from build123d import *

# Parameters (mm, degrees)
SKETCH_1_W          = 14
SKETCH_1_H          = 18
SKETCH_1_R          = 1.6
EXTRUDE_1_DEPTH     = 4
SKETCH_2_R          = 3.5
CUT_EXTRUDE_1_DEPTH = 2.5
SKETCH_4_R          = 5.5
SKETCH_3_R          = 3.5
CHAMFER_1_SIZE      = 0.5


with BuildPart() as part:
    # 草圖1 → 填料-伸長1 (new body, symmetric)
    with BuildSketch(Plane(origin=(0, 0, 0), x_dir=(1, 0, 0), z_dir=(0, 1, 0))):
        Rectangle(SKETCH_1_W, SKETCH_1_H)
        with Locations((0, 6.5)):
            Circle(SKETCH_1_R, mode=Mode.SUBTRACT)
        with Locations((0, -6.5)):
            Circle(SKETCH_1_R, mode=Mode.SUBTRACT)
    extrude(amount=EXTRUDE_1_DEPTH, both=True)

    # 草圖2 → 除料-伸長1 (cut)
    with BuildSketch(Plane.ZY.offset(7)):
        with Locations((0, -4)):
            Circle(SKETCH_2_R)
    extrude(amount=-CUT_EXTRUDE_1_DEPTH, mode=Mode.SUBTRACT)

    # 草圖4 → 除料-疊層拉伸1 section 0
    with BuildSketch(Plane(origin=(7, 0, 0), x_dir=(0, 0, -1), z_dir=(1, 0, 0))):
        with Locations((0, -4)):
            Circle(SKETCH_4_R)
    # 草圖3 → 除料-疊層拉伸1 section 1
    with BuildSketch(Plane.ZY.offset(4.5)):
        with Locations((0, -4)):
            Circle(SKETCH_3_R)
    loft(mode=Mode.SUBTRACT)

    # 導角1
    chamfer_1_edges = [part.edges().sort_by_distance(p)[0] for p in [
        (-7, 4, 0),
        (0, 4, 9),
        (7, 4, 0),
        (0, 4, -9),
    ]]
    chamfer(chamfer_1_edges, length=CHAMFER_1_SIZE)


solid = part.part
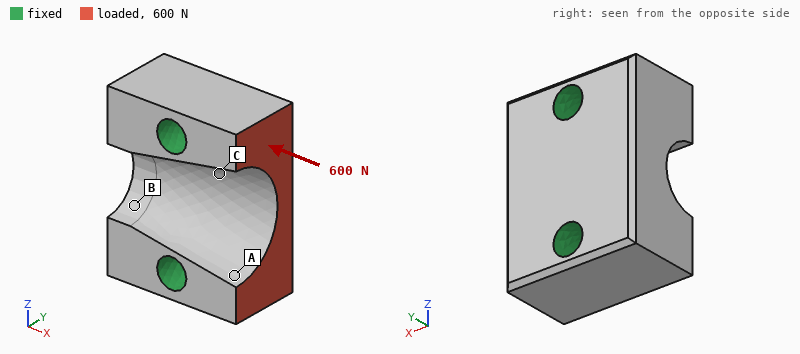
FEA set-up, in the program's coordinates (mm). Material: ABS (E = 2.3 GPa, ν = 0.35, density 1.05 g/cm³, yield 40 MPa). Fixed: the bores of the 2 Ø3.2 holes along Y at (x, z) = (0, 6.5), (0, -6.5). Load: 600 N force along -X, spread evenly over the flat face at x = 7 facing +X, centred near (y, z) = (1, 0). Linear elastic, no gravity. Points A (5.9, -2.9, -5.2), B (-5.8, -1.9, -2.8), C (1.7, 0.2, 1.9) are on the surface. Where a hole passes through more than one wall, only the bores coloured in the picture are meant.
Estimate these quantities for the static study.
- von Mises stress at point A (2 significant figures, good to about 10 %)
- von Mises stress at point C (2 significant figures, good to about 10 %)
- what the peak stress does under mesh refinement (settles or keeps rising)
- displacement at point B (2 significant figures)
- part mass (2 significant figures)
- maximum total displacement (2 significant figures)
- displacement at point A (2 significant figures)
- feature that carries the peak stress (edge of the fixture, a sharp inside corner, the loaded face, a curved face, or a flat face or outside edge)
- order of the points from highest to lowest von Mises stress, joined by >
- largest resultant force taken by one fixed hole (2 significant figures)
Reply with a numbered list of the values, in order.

1. 5.7 MPa
2. 2.1 MPa
3. keeps rising
4. 3.2 µm
5. 1.5 g
6. 20 µm
7. 10 µm
8. edge of the fixture
9. A > C > B
10. 300 N
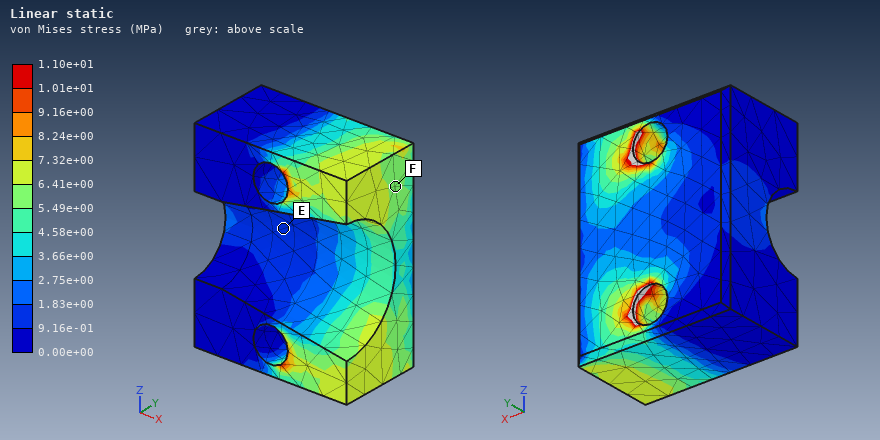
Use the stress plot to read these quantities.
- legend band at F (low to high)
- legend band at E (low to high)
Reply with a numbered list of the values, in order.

1. 5.49e+00 to 6.41e+00 MPa
2. 9.16e-01 to 1.83e+00 MPa
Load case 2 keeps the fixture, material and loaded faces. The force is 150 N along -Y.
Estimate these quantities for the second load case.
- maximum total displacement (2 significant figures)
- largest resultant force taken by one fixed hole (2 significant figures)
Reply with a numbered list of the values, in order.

1. 32 µm
2. 75 N
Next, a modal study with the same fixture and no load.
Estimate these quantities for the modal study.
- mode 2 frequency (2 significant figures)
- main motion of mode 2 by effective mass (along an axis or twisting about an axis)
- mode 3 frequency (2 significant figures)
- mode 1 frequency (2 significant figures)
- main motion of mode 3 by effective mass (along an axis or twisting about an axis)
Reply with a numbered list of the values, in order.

1. 25 kHz
2. along Y
3. 27 kHz
4. 23 kHz
5. along Z
